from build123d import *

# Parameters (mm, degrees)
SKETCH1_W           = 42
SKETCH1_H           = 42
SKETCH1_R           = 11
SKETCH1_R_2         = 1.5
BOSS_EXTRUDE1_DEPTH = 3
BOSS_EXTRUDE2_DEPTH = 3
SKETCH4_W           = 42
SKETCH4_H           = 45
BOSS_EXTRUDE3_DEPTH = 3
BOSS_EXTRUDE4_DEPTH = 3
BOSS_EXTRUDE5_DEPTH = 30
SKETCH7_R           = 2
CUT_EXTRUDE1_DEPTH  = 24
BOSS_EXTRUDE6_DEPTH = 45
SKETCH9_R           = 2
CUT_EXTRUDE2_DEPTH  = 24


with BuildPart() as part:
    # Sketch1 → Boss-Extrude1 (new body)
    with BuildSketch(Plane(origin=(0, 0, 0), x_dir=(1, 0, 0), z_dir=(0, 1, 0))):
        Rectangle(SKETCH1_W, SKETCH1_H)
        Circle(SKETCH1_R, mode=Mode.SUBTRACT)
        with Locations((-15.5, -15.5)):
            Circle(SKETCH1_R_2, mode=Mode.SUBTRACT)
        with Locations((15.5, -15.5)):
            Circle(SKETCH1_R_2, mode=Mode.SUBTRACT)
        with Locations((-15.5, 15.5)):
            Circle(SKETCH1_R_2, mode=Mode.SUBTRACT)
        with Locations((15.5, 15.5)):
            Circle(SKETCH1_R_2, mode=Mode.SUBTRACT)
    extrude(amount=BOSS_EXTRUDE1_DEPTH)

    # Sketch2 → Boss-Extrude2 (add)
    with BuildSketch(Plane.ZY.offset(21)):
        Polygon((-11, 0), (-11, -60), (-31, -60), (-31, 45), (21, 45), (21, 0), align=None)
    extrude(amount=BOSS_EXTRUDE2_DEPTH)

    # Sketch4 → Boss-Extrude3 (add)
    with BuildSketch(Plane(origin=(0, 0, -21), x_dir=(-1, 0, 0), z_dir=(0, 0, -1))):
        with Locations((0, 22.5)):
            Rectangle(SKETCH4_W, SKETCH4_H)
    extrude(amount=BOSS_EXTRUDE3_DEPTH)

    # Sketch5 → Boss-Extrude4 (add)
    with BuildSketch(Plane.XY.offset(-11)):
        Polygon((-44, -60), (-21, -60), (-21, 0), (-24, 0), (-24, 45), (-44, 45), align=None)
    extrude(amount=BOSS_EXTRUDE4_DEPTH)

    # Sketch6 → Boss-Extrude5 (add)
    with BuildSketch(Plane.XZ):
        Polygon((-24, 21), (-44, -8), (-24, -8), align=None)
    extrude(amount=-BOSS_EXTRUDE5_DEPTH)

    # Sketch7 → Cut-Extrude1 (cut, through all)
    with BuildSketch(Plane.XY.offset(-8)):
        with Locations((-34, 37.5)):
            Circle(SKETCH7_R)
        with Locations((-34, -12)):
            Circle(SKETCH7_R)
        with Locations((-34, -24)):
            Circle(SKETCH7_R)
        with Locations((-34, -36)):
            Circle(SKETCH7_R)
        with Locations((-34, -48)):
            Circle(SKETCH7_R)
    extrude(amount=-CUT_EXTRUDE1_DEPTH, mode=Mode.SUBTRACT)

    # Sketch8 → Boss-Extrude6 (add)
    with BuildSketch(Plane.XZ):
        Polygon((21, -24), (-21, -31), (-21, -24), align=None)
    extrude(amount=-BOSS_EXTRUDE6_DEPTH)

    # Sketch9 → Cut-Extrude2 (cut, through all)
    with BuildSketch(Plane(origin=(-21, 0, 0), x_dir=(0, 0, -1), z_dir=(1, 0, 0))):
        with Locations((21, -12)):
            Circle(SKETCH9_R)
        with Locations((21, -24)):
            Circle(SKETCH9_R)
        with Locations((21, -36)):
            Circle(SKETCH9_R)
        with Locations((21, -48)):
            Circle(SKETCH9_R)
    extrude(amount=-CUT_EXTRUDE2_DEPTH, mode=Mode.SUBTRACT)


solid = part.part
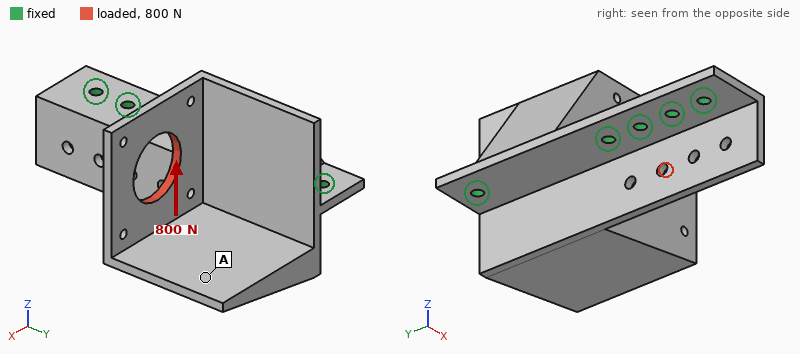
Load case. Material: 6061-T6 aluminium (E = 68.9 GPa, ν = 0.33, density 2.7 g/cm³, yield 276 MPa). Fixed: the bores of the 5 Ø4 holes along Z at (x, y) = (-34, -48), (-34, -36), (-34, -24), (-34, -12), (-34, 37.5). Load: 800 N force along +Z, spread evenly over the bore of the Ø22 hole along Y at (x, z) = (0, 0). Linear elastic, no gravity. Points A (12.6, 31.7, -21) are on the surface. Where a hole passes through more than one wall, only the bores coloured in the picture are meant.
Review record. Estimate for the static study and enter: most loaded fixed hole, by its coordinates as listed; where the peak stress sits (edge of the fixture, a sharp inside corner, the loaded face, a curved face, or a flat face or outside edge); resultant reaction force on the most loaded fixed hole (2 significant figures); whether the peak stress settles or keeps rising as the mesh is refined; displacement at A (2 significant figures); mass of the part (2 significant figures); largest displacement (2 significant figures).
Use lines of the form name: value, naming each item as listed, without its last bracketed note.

most loaded fixed hole, by its coordinates as listed: (-34, 37.5)
where the peak stress sits: edge of the fixture
resultant reaction force on the most loaded fixed hole: 580 N
whether the peak stress settles or keeps rising as the mesh is refined: keeps rising
displacement at A: 0.58 mm
mass of the part: 110 g
largest displacement: 0.73 mm
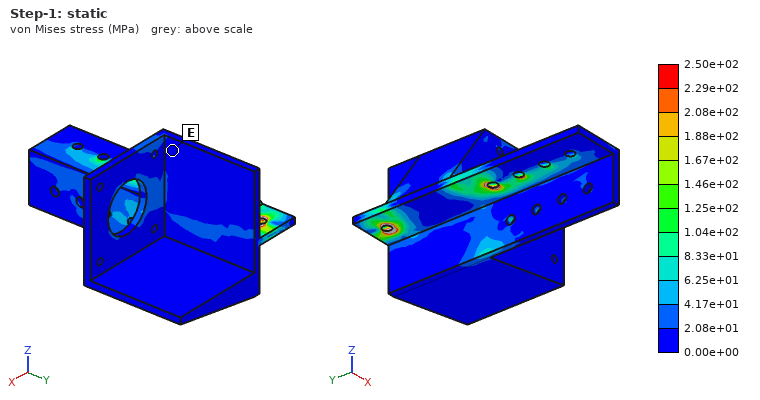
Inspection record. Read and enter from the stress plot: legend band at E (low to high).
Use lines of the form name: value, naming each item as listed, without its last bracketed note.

legend band at E: 0.00e+00 to 2.08e+01 MPa
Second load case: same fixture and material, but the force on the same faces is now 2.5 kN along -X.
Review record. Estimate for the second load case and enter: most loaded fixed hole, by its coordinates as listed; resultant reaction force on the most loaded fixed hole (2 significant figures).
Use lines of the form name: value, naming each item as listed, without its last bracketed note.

most loaded fixed hole, by its coordinates as listed: (-34, -12)
resultant reaction force on the most loaded fixed hole: 2.0 kN
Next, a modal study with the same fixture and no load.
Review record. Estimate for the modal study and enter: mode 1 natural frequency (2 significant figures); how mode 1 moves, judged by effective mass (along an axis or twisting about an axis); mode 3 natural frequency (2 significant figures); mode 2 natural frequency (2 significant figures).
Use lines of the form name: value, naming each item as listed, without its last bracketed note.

mode 1 natural frequency: 860 Hz
how mode 1 moves, judged by effective mass: along Z
mode 3 natural frequency: 3200 Hz
mode 2 natural frequency: 2100 Hz
